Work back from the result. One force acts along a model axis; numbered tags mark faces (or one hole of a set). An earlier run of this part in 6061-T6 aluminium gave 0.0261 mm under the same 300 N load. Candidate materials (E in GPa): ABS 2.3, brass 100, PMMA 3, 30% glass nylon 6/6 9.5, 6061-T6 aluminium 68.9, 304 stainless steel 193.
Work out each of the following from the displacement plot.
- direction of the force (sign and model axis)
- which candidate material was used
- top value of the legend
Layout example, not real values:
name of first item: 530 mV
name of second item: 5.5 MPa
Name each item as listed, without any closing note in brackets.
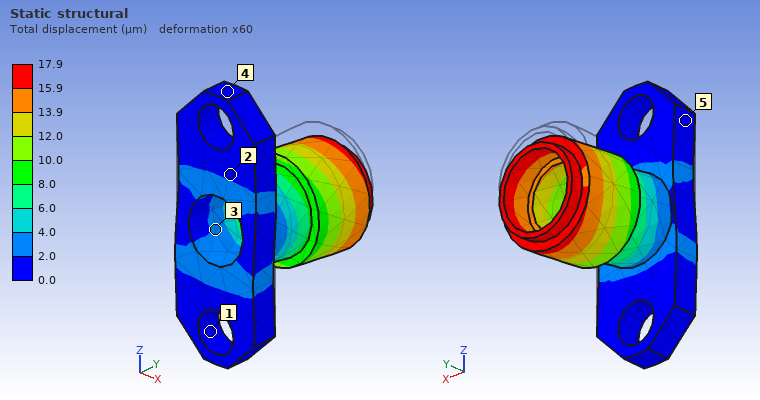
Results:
direction of the force: -Z
which candidate material was used: brass
top value of the legend: 17.9 µm
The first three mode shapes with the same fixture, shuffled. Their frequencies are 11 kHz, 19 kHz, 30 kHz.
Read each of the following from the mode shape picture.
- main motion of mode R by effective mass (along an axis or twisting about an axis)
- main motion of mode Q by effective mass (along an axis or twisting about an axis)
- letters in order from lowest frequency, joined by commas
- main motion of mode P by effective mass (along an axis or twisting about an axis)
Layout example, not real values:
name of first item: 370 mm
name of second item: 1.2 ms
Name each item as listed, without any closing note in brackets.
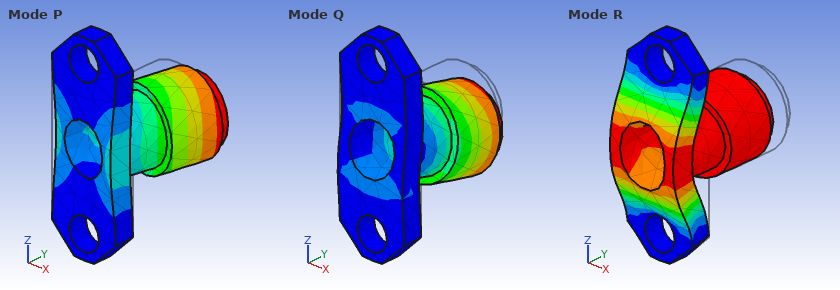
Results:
main motion of mode R by effective mass: along Y
main motion of mode Q by effective mass: along Z
letters in order from lowest frequency, joined by commas: P, Q, R
main motion of mode P by effective mass: along X
